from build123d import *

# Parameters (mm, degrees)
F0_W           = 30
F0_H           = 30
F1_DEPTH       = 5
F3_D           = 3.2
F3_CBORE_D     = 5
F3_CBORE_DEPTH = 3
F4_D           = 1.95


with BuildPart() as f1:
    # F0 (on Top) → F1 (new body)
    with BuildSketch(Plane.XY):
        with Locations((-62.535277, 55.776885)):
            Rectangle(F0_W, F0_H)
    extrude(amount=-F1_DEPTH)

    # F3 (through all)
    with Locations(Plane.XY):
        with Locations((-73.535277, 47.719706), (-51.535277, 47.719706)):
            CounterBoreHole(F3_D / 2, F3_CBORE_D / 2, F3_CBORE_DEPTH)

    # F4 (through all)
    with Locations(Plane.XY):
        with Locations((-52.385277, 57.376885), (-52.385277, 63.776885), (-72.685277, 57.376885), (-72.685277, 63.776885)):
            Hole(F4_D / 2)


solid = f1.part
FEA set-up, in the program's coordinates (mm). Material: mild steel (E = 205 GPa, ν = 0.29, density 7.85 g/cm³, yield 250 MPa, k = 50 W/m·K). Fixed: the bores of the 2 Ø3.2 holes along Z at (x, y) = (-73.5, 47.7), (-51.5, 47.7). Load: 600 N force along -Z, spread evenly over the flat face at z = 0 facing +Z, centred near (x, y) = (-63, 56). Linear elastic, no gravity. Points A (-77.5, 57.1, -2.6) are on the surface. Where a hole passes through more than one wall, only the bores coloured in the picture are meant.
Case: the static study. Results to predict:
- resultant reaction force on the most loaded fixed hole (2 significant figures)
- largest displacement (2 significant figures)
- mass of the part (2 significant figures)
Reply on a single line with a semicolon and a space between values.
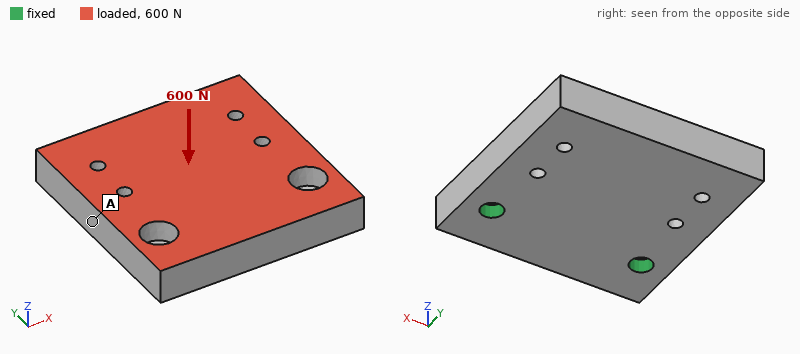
330 N; 34 µm; 34 g
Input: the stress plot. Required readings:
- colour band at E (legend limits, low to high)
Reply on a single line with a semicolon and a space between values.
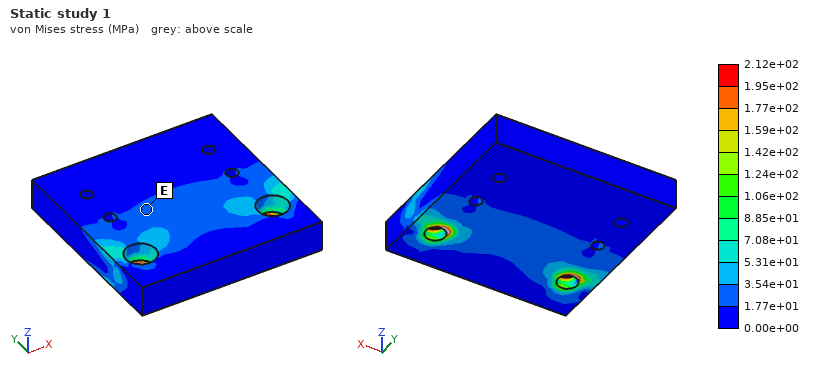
1.77e+01 to 3.54e+01 MPa
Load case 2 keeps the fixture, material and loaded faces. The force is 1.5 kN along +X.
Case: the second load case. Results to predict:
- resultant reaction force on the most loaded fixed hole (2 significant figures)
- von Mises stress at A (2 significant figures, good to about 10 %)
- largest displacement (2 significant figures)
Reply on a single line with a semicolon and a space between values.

960 N; 7.5 MPa; 5.3 µm
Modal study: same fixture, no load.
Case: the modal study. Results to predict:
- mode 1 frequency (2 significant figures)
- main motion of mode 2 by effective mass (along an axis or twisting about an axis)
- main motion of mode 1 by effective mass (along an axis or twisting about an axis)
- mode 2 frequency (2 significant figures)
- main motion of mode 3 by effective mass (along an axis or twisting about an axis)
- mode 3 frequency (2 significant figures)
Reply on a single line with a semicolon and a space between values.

4400 Hz; twisting about Y; along Z; 12 kHz; along X; 21 kHz
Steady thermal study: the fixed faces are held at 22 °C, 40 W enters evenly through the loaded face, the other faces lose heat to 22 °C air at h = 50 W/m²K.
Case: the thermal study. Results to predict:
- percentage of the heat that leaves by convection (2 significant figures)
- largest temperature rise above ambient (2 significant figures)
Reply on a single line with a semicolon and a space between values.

9.8 %; 71 K
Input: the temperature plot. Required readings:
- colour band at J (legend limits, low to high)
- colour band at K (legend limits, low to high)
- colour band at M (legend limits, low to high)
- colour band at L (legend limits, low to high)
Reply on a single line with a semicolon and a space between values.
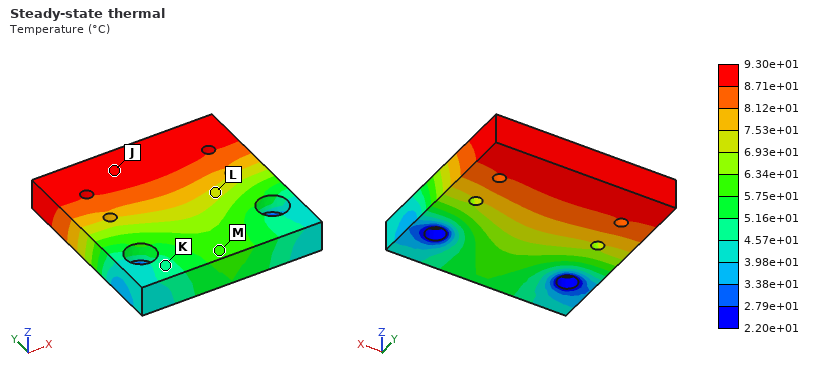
8.71e+01 to 9.30e+01 °C; 4.57e+01 to 5.16e+01 °C; 5.75e+01 to 6.34e+01 °C; 6.93e+01 to 7.53e+01 °C
